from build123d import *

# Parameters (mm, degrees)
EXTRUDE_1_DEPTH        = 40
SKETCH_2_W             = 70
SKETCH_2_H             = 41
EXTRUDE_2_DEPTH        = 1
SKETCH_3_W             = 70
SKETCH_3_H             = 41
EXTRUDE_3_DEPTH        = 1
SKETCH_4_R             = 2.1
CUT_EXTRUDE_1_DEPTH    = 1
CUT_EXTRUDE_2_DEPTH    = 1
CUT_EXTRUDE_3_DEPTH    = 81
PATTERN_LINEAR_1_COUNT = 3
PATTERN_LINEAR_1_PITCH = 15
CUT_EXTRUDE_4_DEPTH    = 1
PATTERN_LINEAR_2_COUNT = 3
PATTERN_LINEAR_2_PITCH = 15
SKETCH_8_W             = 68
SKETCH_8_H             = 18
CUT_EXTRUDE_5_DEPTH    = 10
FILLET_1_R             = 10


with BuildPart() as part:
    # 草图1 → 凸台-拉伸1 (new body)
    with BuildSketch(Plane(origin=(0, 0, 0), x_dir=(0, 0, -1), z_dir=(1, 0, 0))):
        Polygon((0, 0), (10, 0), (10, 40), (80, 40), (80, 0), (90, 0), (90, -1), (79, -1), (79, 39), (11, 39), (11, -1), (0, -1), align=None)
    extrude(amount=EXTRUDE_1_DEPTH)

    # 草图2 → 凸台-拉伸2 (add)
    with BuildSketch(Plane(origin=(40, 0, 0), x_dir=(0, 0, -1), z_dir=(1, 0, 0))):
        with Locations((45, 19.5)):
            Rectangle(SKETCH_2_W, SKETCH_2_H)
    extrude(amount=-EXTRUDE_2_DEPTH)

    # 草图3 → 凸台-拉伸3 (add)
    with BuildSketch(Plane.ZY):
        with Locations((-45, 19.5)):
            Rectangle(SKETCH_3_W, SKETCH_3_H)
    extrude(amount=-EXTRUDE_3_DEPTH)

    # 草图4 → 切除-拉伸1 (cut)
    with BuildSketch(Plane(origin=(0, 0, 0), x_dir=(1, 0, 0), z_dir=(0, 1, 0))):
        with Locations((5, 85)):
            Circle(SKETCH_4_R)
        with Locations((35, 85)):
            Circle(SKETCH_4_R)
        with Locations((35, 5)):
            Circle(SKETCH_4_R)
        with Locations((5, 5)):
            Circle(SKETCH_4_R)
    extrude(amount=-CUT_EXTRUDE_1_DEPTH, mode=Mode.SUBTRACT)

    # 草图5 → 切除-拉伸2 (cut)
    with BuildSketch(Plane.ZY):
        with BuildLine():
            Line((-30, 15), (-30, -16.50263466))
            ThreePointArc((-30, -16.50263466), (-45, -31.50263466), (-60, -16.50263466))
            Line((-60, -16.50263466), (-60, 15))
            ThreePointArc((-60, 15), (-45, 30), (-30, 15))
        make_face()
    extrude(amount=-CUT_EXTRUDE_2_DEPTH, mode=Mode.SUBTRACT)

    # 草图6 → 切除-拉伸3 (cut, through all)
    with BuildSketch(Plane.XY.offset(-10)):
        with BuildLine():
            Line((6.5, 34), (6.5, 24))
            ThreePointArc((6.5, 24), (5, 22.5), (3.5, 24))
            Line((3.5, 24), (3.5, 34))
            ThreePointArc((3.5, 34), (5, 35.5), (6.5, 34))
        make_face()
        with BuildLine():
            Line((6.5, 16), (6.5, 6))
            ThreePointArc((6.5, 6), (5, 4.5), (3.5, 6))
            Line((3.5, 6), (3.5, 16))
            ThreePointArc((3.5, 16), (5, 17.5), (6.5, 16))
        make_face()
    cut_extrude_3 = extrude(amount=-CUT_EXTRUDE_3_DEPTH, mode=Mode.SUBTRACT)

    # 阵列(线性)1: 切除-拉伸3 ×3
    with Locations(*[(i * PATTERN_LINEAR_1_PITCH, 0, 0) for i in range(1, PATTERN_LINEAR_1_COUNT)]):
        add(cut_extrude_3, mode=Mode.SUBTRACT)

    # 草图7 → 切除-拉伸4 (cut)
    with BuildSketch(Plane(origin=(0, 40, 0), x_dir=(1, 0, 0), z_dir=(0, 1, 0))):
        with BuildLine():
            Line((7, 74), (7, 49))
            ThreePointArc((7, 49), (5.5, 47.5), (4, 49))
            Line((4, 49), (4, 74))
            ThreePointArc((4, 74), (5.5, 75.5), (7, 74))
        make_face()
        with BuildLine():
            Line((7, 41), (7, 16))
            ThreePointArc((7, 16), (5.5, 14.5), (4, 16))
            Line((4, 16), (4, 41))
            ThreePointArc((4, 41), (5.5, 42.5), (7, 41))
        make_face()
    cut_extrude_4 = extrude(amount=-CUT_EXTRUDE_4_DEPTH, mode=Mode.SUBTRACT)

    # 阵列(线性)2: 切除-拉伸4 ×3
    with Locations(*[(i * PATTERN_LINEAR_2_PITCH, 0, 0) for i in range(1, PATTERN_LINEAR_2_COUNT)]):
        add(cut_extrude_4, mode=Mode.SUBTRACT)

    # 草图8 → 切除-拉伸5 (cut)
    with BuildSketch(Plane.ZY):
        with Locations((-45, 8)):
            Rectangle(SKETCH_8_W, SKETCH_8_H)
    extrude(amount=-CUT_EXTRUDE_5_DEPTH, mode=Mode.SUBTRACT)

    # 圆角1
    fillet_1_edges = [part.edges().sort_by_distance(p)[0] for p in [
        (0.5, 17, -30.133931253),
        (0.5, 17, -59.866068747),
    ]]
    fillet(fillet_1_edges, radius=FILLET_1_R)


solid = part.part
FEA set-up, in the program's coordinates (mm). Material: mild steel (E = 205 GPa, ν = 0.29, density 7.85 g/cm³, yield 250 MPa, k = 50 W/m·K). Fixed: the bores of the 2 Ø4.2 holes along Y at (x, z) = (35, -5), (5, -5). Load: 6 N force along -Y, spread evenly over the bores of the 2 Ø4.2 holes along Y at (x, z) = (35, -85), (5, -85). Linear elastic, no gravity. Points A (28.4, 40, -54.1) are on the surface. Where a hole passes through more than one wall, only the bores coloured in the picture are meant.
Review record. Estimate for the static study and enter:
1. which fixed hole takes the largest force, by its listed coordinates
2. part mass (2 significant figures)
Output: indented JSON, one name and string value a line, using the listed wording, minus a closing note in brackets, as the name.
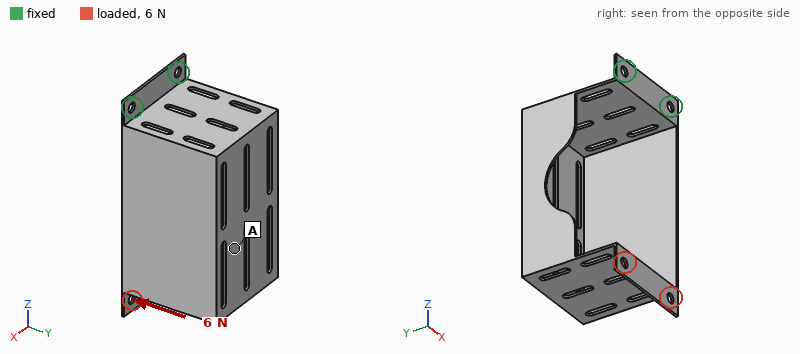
{
  "which fixed hole takes the largest force, by its listed coordinates": "(35, -5)",
  "part mass": "76 g"
}
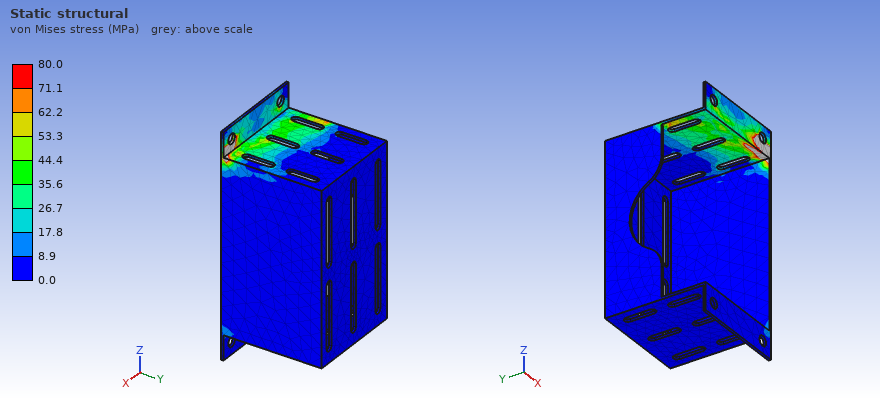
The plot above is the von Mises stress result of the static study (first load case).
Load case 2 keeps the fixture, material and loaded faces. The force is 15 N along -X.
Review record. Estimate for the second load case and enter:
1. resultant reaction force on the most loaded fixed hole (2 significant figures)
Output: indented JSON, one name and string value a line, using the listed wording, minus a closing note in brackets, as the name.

{
  "resultant reaction force on the most loaded fixed hole": "35 N"
}
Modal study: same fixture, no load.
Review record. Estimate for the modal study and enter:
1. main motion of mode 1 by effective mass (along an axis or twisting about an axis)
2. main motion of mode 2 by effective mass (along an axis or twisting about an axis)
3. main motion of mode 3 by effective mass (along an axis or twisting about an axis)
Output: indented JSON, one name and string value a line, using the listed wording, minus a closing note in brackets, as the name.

{
  "main motion of mode 1 by effective mass": "along Y",
  "main motion of mode 2 by effective mass": "along X",
  "main motion of mode 3 by effective mass": "along Z"
}
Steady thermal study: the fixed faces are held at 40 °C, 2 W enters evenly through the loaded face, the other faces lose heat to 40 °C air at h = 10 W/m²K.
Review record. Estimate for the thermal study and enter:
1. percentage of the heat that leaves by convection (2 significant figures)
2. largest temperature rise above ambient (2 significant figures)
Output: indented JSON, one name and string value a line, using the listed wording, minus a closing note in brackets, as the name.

{
  "percentage of the heat that leaves by convection": "89 %",
  "largest temperature rise above ambient": "43 K"
}
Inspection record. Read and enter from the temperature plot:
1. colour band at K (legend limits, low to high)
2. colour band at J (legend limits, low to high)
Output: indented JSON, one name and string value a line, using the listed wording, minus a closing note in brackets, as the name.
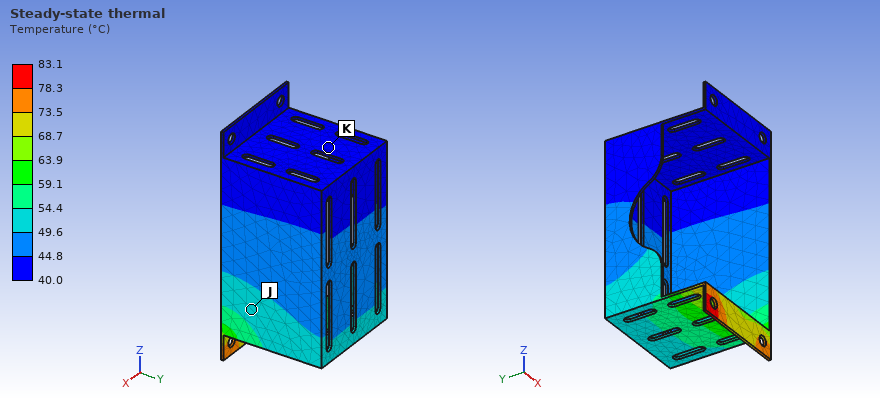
{
  "colour band at K": "40.0 to 44.8 °C",
  "colour band at J": "49.6 to 54.4 °C"
}
